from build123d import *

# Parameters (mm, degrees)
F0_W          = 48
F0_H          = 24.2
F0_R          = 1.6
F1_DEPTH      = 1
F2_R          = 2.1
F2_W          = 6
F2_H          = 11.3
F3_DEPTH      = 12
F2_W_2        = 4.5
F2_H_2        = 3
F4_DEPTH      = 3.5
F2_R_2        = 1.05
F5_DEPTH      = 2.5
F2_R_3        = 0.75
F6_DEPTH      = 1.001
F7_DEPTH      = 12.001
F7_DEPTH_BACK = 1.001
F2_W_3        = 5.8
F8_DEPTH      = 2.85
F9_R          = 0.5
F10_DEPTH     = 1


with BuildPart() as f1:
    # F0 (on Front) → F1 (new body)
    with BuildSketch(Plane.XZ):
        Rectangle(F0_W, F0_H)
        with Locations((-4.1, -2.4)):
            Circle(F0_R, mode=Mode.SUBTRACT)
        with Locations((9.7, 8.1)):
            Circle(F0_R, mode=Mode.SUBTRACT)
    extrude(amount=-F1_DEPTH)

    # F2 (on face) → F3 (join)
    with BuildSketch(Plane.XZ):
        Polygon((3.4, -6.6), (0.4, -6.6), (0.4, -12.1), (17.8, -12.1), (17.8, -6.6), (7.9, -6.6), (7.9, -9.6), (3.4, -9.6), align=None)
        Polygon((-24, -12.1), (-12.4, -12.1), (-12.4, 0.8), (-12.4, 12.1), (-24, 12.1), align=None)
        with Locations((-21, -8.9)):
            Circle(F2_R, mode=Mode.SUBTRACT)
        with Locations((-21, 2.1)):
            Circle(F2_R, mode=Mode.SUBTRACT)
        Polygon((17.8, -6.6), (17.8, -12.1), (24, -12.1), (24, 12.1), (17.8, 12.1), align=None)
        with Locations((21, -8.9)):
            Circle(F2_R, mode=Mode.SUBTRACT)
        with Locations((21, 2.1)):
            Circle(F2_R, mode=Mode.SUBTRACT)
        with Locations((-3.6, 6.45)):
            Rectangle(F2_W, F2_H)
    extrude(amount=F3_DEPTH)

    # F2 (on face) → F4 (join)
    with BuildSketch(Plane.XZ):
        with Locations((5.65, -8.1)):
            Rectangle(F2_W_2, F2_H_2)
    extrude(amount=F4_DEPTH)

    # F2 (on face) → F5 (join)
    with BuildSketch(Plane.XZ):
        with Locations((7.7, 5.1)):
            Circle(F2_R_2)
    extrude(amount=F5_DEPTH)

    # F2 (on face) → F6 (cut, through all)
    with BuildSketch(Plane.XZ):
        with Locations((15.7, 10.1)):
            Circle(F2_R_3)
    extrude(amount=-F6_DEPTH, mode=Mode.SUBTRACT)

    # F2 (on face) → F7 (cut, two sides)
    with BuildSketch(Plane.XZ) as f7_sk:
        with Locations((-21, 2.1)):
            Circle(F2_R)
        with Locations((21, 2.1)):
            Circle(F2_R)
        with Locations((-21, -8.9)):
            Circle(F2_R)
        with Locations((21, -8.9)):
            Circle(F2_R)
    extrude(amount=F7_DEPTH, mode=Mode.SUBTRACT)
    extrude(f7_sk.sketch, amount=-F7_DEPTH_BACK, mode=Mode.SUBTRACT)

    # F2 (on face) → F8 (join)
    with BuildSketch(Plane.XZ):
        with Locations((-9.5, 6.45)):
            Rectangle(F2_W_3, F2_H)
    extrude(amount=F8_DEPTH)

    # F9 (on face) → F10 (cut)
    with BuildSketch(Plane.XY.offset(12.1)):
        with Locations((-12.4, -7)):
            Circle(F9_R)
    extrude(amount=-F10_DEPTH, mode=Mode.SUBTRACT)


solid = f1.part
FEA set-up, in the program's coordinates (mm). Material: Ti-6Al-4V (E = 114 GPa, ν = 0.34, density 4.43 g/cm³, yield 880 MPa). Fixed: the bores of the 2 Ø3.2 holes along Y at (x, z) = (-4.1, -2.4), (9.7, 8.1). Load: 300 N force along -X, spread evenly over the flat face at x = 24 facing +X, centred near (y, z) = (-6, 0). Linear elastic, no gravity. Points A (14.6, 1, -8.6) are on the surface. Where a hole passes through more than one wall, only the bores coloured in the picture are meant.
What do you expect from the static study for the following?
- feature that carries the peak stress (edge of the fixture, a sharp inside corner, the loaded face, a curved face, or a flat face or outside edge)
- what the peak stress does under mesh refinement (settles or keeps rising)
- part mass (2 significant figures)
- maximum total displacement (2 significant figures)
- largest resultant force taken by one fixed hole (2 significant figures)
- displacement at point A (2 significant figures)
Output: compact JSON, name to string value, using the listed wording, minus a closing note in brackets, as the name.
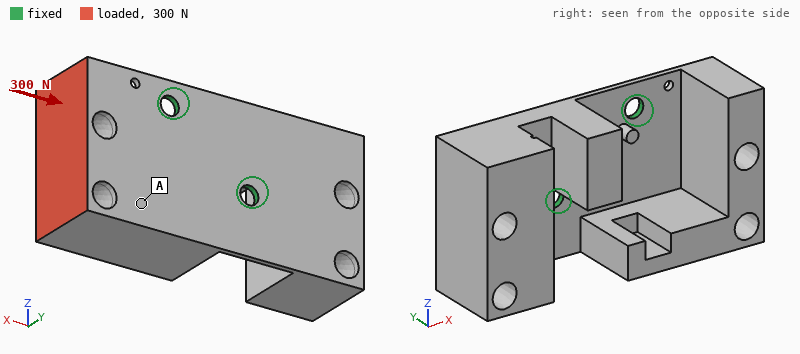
{"feature that carries the peak stress": "edge of the fixture", "what the peak stress does under mesh refinement": "keeps rising", "part mass": "34 g", "maximum total displacement": "0.59 mm", "largest resultant force taken by one fixed hole": "180 N", "displacement at point A": "0.29 mm"}
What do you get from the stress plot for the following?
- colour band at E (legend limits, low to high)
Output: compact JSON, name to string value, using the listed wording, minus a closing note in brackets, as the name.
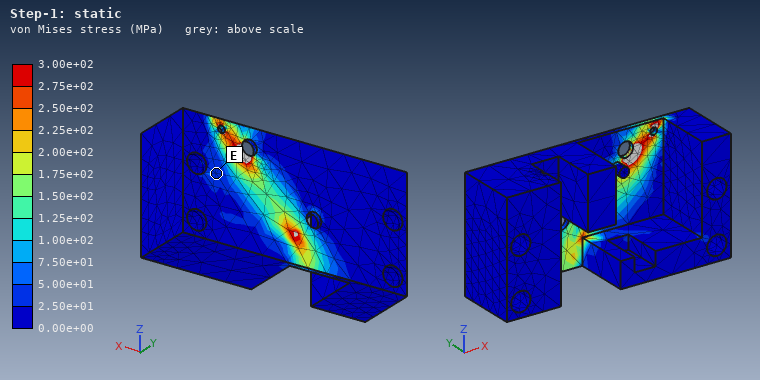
{"colour band at E": "2.50e+01 to 5.00e+01 MPa"}
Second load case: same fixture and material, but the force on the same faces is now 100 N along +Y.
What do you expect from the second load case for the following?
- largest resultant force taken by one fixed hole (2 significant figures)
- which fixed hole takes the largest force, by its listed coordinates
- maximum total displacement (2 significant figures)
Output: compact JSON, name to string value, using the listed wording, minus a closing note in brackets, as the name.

{"largest resultant force taken by one fixed hole": "140 N", "which fixed hole takes the largest force, by its listed coordinates": "(9.7, 8.1)", "maximum total displacement": "0.61 mm"}
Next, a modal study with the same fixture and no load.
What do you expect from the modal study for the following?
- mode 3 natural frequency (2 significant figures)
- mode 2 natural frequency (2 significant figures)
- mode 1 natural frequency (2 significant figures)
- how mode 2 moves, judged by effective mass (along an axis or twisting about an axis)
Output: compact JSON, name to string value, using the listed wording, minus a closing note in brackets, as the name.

{"mode 3 natural frequency": "1800 Hz", "mode 2 natural frequency": "1000 Hz", "mode 1 natural frequency": "780 Hz", "how mode 2 moves, judged by effective mass": "along Y"}
